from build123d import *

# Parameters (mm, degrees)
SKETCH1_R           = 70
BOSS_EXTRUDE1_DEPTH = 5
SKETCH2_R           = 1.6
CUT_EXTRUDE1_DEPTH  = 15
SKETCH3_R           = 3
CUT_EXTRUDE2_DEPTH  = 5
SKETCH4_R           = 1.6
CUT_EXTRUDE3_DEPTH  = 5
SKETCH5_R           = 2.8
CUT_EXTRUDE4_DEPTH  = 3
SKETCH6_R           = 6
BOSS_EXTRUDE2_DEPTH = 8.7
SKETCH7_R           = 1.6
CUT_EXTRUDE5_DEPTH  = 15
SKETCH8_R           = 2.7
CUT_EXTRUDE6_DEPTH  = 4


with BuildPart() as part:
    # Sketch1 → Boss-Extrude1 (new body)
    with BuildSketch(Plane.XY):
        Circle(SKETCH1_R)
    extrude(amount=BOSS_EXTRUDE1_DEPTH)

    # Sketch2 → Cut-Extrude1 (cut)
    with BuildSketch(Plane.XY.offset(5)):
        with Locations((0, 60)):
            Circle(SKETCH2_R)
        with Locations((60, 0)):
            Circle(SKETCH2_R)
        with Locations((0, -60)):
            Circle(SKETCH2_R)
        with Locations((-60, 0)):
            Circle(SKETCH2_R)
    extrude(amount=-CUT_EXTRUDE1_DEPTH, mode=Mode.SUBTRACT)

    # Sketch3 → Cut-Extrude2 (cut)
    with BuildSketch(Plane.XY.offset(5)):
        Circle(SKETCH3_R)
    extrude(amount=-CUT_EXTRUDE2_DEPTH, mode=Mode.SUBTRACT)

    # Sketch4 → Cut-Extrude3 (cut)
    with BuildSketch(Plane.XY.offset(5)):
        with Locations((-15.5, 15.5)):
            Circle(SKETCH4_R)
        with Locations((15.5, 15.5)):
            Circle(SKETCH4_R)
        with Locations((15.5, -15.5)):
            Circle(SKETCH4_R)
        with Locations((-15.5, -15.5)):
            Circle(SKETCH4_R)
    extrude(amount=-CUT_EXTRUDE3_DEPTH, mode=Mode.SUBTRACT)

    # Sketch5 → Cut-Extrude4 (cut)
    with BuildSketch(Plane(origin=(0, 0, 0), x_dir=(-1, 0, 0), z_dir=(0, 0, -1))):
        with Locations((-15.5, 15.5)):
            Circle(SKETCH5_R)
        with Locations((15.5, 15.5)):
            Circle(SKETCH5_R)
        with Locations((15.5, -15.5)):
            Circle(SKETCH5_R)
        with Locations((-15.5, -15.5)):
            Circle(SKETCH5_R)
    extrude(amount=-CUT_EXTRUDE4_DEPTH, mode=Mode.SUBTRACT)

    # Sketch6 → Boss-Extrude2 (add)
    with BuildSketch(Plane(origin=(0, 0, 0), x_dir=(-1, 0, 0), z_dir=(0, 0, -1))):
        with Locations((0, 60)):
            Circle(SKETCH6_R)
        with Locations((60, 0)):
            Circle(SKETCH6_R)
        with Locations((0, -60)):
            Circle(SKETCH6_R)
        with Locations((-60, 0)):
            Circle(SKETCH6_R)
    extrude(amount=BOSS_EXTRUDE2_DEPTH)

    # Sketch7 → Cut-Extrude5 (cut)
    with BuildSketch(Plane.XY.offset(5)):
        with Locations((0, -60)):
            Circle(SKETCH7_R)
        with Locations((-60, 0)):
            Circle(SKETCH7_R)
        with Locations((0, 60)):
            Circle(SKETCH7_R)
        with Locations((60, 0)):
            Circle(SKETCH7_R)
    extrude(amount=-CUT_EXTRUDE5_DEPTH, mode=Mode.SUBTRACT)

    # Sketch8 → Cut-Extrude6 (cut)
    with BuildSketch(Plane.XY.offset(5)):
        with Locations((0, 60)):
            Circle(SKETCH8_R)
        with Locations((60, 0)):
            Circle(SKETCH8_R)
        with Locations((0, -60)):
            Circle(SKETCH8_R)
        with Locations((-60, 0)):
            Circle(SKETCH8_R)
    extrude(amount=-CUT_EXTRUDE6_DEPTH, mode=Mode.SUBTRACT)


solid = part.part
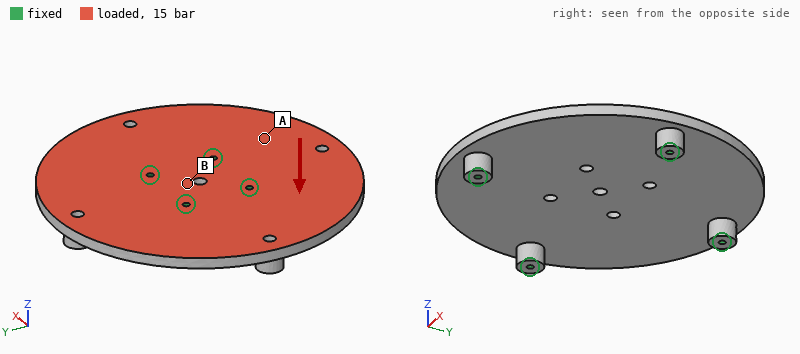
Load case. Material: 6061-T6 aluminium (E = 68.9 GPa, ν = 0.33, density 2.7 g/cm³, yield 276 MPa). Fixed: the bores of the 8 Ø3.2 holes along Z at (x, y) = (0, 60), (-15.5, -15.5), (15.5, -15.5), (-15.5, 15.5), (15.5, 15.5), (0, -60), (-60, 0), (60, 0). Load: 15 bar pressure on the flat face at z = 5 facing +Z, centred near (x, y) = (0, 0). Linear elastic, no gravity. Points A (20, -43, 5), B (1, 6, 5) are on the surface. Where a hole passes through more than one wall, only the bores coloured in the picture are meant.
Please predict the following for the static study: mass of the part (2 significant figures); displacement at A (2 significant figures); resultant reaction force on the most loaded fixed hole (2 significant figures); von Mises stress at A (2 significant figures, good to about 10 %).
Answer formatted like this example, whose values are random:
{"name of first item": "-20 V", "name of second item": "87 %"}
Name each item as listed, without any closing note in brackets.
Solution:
{"mass of the part": "220 g", "displacement at A": "0.14 mm", "resultant reaction force on the most loaded fixed hole": "3.8 kN", "von Mises stress at A": "72 MPa"}
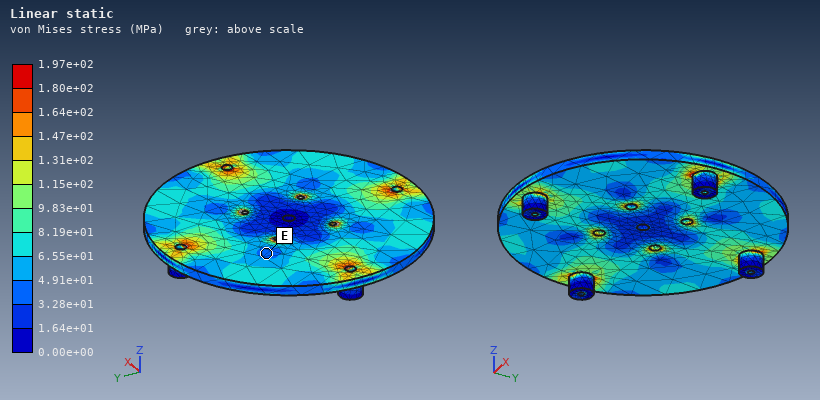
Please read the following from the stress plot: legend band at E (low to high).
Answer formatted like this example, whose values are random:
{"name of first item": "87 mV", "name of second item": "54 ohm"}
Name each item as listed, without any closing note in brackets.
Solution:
{"legend band at E": "3.28e+01 to 4.91e+01 MPa"}
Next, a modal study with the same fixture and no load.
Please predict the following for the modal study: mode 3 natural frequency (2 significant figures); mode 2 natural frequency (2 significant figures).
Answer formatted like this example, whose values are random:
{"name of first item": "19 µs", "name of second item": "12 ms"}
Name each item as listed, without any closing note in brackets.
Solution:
{"mode 3 natural frequency": "3300 Hz", "mode 2 natural frequency": "3300 Hz"}
